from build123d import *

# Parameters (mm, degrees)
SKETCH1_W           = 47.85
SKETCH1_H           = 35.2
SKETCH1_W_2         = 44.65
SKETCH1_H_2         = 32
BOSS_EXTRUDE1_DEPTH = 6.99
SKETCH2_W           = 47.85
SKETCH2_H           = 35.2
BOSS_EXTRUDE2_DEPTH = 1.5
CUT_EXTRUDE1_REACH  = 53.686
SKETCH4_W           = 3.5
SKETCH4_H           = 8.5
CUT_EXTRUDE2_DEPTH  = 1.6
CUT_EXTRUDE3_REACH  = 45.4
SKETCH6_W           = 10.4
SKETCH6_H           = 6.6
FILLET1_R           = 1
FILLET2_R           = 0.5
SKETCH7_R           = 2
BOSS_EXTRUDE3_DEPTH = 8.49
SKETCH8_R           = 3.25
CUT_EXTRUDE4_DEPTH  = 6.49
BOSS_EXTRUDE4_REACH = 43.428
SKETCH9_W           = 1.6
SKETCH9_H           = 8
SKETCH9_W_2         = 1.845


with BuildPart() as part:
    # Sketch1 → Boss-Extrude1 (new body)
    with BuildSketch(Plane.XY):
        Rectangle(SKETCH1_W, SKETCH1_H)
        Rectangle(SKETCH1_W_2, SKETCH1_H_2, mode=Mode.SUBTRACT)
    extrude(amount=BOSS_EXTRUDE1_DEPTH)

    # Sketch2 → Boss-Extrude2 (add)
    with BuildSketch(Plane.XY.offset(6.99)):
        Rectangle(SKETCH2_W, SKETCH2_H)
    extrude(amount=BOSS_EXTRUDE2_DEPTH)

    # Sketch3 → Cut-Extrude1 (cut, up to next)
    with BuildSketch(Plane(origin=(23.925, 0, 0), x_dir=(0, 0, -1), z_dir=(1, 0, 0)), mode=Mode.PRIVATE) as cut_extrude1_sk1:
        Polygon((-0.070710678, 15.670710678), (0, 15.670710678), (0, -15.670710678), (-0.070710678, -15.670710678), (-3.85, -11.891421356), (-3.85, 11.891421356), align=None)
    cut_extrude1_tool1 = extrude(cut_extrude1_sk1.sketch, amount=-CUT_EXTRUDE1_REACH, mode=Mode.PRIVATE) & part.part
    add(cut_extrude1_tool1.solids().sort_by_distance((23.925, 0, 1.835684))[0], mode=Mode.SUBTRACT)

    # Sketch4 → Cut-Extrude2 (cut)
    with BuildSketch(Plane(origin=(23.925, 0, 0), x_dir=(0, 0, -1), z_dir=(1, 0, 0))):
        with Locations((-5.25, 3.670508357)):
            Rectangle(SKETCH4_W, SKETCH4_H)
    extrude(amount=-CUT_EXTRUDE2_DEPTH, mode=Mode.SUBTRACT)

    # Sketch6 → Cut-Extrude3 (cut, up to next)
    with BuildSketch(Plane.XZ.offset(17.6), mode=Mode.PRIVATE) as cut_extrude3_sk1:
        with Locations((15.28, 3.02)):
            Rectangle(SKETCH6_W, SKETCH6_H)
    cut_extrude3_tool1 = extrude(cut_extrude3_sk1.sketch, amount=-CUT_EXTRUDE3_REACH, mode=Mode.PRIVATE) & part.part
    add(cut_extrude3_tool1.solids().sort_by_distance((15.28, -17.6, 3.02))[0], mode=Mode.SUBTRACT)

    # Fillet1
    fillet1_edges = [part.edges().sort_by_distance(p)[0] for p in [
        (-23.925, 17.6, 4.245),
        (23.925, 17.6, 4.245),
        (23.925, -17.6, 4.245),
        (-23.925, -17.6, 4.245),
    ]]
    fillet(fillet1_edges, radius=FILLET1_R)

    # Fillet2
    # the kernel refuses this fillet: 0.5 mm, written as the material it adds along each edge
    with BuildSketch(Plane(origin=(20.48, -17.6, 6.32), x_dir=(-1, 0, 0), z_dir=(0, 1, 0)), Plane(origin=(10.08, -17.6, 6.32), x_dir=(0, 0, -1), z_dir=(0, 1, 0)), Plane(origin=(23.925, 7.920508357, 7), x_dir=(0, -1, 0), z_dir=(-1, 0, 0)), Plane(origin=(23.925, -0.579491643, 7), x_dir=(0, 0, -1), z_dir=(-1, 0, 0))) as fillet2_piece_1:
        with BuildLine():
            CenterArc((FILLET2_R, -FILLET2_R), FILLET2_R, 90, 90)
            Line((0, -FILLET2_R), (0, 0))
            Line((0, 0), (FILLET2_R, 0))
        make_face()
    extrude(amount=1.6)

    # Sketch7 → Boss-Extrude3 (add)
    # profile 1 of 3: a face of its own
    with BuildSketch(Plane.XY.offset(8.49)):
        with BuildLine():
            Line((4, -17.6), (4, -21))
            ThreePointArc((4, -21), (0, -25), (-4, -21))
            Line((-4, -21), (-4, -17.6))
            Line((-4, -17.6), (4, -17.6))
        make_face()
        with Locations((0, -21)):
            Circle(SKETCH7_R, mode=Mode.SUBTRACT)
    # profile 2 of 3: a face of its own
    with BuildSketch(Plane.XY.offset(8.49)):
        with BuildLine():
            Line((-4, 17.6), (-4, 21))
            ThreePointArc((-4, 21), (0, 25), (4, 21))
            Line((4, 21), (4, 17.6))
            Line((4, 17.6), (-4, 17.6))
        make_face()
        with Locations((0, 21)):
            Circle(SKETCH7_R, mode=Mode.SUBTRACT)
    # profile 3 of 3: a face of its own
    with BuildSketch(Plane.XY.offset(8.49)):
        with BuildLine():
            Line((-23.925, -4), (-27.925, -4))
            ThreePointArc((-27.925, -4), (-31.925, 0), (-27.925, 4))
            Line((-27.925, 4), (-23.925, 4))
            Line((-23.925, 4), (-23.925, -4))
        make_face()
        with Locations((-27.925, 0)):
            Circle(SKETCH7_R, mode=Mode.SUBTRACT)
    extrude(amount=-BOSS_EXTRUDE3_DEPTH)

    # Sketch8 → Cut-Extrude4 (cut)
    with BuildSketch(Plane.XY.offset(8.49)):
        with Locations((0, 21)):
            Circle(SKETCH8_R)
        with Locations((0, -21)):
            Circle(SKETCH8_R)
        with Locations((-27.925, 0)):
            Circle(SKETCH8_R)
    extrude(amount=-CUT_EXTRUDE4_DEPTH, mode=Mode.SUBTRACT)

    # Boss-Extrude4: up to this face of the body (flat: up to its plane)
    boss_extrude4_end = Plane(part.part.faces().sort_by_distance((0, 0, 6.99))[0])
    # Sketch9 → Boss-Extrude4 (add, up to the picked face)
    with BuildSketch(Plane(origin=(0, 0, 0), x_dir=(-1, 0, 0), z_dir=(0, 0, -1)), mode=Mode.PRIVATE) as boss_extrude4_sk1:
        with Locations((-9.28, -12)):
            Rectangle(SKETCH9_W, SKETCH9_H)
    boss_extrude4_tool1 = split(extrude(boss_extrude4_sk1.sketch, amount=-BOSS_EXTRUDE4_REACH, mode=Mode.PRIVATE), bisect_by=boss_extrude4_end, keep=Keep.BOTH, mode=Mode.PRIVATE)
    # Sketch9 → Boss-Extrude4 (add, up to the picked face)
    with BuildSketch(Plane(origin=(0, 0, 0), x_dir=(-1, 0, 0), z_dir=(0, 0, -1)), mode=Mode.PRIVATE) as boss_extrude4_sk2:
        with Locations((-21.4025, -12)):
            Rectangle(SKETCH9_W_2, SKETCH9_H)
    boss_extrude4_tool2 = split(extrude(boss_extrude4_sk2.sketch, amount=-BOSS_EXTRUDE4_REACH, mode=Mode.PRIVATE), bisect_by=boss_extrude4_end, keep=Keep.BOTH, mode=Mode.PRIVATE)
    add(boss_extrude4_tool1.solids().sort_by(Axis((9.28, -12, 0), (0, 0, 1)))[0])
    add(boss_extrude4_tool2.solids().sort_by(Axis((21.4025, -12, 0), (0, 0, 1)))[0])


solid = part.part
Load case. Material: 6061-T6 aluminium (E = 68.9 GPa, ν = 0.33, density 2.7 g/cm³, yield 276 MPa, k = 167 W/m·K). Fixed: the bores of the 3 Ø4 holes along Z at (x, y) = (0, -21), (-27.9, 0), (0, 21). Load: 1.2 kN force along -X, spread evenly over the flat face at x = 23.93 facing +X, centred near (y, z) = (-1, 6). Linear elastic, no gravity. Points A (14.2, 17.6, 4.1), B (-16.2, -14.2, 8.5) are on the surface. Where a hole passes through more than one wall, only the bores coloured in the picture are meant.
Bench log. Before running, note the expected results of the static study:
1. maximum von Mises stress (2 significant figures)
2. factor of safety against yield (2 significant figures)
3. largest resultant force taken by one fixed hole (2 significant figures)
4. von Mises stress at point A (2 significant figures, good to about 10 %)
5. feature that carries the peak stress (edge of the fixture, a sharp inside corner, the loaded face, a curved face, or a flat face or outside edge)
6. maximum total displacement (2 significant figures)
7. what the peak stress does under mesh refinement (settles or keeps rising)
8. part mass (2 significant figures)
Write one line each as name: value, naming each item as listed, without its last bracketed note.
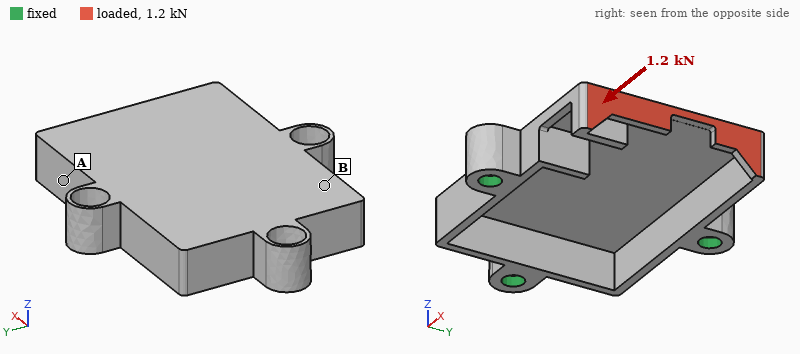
maximum von Mises stress: 420 MPa
factor of safety against yield: 0.66
largest resultant force taken by one fixed hole: 480 N
von Mises stress at point A: 43 MPa
feature that carries the peak stress: a curved face
maximum total displacement: 0.33 mm
what the peak stress does under mesh refinement: settles
part mass: 13 g
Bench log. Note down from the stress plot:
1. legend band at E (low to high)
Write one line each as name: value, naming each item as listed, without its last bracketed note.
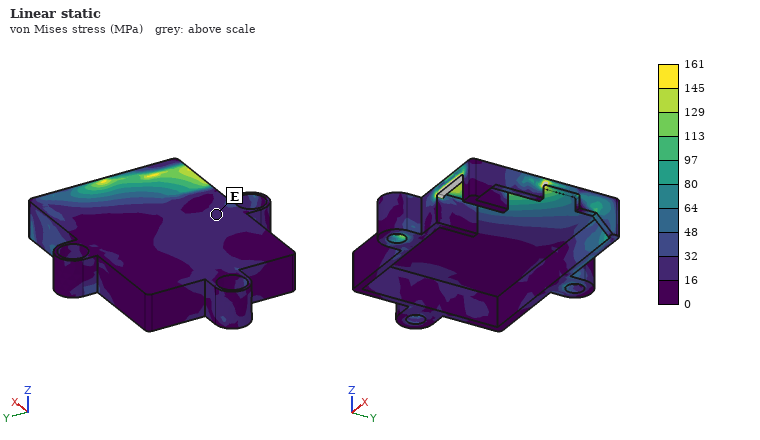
legend band at E: 16 to 32 MPa
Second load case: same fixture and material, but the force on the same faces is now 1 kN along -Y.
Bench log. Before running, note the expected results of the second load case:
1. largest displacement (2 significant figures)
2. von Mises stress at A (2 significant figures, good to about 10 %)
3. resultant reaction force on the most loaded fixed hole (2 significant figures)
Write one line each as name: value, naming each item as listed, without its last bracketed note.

largest displacement: 0.30 mm
von Mises stress at A: 81 MPa
resultant reaction force on the most loaded fixed hole: 780 N
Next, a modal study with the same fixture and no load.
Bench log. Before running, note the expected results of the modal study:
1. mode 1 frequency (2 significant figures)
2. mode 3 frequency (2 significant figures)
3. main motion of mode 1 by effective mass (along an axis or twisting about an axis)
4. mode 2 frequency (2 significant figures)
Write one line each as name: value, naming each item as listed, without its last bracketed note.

mode 1 frequency: 3300 Hz
mode 3 frequency: 7400 Hz
main motion of mode 1 by effective mass: along Z
mode 2 frequency: 5600 Hz
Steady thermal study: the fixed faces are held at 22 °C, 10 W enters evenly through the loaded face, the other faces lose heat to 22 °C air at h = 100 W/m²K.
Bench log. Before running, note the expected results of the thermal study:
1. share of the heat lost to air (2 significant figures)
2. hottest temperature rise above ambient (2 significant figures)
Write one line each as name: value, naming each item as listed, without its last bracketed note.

share of the heat lost to air: 38 %
hottest temperature rise above ambient: 23 K
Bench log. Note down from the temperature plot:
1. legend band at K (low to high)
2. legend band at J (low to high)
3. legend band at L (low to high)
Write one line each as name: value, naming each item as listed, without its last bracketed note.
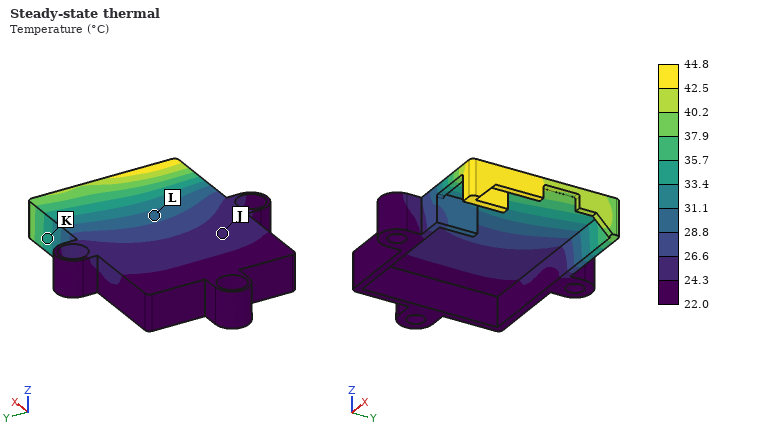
legend band at K: 33.4 to 35.7 °C
legend band at J: 24.3 to 26.6 °C
legend band at L: 28.8 to 31.1 °C
